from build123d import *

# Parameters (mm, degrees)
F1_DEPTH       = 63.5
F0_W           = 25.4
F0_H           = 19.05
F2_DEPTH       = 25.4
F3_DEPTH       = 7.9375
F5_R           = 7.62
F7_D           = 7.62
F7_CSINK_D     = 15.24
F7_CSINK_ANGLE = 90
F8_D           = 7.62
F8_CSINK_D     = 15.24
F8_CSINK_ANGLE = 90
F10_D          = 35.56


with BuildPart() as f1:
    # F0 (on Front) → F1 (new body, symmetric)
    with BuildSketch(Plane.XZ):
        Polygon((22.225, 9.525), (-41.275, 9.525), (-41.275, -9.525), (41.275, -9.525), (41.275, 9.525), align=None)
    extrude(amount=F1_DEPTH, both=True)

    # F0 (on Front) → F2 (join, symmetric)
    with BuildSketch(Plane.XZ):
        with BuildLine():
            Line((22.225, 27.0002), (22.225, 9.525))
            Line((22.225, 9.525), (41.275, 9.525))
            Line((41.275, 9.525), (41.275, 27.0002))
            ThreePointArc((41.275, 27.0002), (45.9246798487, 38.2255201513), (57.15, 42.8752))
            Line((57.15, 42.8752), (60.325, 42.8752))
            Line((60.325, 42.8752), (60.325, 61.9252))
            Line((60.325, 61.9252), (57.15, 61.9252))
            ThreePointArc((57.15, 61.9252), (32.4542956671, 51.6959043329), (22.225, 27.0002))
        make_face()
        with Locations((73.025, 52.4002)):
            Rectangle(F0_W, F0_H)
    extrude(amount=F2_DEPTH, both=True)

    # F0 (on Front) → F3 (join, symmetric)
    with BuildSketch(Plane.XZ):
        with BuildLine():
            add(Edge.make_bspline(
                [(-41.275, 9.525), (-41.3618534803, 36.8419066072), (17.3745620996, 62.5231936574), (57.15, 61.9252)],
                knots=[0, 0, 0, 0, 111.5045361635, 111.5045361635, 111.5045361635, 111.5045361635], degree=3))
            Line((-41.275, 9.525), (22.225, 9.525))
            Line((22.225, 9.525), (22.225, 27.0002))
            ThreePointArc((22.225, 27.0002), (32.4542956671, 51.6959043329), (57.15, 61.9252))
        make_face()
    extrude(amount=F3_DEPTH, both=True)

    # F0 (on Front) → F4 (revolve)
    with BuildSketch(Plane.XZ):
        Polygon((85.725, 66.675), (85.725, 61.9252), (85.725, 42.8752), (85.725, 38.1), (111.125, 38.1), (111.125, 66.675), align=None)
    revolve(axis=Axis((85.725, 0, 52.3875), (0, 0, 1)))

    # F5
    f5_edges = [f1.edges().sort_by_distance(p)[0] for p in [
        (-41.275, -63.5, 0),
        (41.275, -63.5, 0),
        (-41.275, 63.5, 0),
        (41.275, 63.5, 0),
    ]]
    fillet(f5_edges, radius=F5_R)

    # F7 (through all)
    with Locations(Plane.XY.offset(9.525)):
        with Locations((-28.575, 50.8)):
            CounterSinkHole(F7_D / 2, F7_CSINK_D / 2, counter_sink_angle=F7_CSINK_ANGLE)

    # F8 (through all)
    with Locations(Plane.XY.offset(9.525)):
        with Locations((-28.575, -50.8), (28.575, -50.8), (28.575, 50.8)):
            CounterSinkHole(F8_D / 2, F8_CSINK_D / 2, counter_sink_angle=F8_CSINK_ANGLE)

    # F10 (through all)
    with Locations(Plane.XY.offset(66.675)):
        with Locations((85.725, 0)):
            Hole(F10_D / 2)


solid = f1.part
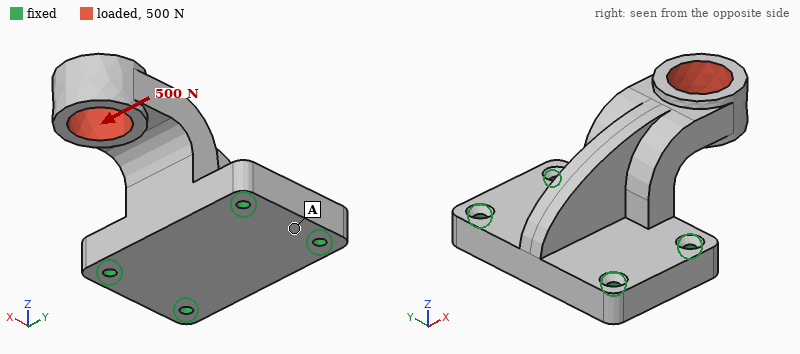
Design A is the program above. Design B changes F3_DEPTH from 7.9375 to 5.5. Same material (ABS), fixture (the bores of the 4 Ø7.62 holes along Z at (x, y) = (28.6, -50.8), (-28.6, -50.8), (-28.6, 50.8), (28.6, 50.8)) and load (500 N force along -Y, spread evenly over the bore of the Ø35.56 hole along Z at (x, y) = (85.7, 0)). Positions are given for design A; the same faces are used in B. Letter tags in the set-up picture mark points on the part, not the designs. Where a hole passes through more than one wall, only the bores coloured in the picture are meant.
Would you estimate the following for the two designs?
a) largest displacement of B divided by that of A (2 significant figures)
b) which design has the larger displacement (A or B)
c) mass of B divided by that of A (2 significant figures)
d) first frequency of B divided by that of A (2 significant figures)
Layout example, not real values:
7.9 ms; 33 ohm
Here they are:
1.1; B; 0.97; 0.97
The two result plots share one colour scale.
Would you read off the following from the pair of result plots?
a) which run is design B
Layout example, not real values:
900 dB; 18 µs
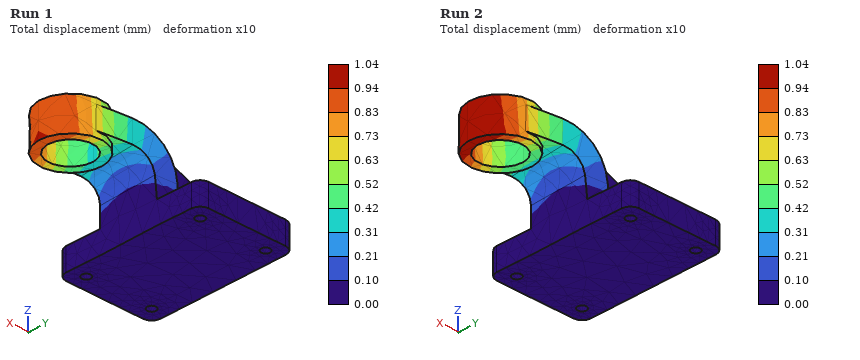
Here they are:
Run 2
